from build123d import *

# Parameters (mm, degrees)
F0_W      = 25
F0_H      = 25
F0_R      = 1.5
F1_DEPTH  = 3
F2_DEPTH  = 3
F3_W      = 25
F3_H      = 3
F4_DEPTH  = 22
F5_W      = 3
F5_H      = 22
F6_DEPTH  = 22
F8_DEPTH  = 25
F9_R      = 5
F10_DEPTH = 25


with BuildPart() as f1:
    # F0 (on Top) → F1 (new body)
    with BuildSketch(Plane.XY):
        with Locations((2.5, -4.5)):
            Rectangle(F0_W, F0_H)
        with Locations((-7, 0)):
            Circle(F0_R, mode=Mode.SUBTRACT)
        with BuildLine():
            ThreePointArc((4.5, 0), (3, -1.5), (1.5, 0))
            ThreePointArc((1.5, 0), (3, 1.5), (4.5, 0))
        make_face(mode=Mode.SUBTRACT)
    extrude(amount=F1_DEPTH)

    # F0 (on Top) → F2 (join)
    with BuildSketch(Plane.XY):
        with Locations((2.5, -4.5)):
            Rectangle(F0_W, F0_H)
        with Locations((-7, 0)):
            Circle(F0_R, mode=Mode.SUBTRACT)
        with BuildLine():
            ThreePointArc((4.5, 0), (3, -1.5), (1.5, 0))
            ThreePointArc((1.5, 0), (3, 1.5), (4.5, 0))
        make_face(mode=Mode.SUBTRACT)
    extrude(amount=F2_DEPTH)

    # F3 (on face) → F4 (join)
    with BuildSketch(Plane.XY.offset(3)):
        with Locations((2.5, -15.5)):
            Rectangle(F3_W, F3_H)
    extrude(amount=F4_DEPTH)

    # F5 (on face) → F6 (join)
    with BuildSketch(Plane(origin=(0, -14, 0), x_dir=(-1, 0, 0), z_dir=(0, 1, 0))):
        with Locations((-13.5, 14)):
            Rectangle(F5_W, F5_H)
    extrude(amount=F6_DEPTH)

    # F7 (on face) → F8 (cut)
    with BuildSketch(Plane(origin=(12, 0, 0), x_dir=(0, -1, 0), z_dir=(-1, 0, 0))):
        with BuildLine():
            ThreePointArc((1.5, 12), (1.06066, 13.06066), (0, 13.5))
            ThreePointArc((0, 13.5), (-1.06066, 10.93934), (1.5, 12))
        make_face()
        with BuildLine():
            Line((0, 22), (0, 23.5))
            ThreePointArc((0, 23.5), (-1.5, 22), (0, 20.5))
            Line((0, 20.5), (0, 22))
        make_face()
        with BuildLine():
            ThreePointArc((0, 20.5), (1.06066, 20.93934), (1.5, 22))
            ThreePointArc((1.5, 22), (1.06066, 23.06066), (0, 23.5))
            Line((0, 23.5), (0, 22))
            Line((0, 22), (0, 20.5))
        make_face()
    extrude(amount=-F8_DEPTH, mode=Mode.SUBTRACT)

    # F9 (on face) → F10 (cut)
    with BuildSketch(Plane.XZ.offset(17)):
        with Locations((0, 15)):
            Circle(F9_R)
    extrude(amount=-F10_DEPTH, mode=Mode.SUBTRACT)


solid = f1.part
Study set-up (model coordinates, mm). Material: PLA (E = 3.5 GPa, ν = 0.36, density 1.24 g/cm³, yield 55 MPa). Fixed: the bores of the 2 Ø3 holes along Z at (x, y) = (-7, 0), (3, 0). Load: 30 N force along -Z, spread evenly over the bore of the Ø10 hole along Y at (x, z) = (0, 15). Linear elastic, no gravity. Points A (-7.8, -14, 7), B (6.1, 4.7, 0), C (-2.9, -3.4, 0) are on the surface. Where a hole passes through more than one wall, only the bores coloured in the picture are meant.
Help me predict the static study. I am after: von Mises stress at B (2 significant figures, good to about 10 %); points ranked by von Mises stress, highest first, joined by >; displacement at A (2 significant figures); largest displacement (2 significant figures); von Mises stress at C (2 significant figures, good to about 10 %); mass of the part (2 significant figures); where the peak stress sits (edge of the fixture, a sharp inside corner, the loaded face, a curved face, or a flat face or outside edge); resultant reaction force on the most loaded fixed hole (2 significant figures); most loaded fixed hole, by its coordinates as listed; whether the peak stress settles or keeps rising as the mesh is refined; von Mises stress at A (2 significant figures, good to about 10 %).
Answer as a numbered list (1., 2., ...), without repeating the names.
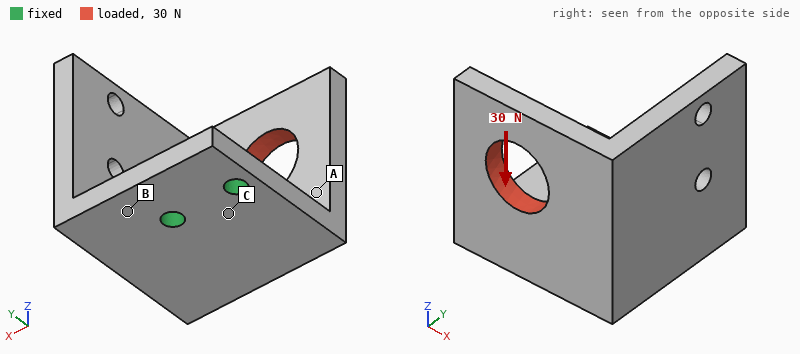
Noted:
1. 4.2 MPa
2. C > B > A
3. 0.15 mm
4. 0.32 mm
5. 7.0 MPa
6. 5.8 g
7. edge of the fixture
8. 18 N
9. (3, 0)
10. keeps rising
11. 2.0 MPa
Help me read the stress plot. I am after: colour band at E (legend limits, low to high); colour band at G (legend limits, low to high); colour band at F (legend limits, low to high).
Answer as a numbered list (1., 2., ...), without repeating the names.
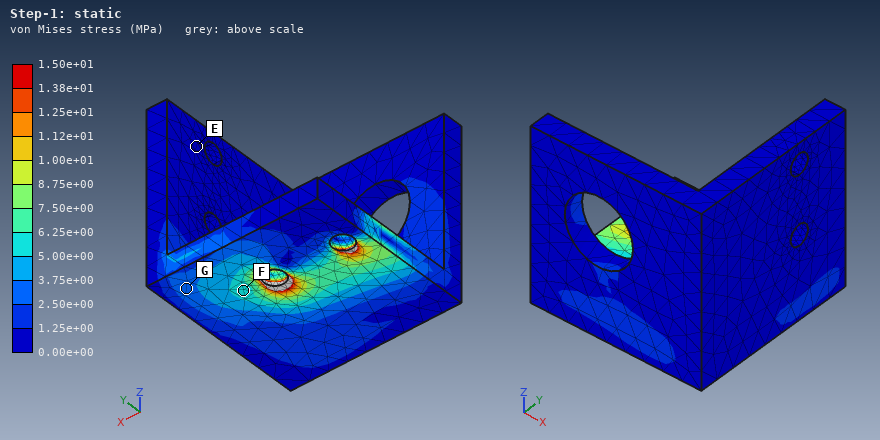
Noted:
1. 0.00e+00 to 1.25e+00 MPa
2. 2.50e+00 to 3.75e+00 MPa
3. 5.00e+00 to 6.25e+00 MPa
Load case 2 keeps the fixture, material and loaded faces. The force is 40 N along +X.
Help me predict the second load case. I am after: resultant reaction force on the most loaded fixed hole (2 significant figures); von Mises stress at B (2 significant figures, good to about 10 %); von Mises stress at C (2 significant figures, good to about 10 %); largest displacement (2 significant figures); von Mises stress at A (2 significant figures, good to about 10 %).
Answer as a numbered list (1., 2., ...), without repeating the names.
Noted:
1. 65 N
2. 6.8 MPa
3. 4.2 MPa
4. 0.45 mm
5. 5.3 MPa
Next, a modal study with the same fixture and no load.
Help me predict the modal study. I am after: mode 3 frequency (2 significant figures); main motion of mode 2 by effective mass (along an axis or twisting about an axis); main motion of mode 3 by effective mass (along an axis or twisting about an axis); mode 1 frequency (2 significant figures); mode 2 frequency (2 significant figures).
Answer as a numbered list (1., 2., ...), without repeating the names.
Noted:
1. 2300 Hz
2. along X
3. along Z
4. 790 Hz
5. 1000 Hz
